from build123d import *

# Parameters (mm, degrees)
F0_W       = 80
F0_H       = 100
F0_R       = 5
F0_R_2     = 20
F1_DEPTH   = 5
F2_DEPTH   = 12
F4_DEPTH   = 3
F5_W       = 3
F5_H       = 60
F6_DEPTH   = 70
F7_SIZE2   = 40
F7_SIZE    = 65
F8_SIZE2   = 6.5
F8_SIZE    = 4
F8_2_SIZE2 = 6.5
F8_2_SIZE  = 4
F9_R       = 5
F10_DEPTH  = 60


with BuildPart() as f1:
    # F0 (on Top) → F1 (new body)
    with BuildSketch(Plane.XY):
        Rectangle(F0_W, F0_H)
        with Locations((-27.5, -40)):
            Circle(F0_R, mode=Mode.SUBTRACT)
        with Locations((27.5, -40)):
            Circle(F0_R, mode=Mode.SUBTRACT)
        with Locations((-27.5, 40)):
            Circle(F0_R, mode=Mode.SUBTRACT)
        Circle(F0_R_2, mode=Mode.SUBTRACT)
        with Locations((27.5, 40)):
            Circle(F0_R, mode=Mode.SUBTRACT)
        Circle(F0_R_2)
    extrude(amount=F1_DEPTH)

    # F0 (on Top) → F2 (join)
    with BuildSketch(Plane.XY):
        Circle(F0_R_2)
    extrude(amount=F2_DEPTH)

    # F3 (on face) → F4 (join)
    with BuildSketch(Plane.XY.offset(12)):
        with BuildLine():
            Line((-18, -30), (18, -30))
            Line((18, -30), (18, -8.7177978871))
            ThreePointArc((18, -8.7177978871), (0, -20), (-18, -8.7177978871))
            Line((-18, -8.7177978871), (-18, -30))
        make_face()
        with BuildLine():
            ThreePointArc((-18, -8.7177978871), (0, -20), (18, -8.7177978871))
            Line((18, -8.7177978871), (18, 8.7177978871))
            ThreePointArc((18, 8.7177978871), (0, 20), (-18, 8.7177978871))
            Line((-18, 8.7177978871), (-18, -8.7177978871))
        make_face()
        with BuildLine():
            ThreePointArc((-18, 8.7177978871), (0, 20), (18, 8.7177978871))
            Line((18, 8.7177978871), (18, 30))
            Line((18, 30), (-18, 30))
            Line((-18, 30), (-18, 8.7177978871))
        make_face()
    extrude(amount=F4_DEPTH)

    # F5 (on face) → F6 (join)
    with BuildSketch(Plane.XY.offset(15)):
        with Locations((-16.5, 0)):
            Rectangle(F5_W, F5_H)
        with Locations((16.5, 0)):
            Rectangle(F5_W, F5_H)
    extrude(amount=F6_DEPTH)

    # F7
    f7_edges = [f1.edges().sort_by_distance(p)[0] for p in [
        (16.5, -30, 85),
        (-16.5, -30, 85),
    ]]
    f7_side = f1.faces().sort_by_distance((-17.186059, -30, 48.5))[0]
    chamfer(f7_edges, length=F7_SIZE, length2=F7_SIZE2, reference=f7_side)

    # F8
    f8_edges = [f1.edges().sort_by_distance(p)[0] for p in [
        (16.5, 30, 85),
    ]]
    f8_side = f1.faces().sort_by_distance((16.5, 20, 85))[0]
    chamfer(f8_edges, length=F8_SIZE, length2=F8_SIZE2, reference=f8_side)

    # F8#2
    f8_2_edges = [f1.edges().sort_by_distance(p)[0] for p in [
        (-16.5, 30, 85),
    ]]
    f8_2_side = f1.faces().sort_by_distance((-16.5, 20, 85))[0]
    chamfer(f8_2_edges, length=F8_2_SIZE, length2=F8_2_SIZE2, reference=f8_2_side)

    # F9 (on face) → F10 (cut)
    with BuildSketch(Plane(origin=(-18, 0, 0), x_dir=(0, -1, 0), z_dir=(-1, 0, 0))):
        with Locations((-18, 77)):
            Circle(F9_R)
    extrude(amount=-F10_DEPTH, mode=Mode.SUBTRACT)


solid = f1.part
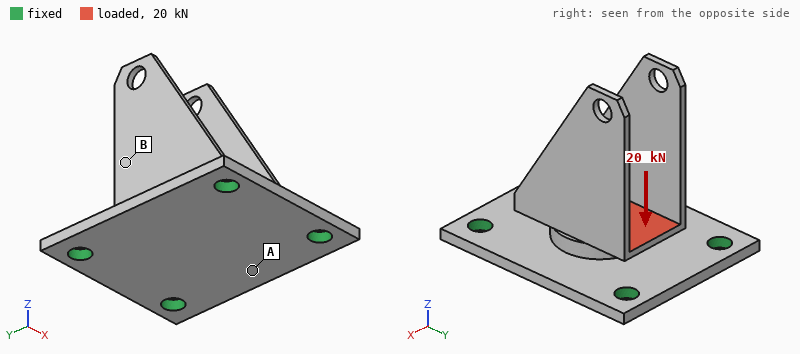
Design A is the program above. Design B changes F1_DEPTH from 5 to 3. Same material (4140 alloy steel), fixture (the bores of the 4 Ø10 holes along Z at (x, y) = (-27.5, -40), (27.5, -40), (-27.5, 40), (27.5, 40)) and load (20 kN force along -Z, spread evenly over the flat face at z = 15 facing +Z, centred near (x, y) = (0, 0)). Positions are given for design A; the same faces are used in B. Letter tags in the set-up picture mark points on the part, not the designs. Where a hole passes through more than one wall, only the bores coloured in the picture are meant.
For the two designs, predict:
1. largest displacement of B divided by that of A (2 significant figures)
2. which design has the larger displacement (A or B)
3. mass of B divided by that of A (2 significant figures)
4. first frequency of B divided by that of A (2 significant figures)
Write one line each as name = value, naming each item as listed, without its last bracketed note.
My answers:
largest displacement of B divided by that of A = 3.2
which design has the larger displacement = B
mass of B divided by that of A = 0.82
first frequency of B divided by that of A = 0.91
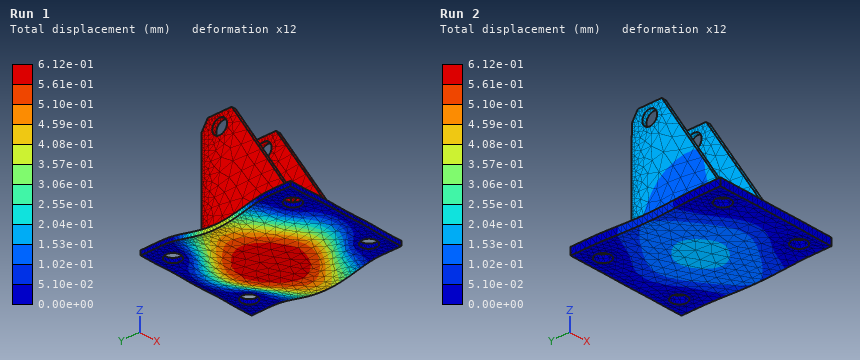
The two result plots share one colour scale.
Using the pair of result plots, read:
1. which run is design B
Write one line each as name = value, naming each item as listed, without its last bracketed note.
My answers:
which run is design B = Run 1
